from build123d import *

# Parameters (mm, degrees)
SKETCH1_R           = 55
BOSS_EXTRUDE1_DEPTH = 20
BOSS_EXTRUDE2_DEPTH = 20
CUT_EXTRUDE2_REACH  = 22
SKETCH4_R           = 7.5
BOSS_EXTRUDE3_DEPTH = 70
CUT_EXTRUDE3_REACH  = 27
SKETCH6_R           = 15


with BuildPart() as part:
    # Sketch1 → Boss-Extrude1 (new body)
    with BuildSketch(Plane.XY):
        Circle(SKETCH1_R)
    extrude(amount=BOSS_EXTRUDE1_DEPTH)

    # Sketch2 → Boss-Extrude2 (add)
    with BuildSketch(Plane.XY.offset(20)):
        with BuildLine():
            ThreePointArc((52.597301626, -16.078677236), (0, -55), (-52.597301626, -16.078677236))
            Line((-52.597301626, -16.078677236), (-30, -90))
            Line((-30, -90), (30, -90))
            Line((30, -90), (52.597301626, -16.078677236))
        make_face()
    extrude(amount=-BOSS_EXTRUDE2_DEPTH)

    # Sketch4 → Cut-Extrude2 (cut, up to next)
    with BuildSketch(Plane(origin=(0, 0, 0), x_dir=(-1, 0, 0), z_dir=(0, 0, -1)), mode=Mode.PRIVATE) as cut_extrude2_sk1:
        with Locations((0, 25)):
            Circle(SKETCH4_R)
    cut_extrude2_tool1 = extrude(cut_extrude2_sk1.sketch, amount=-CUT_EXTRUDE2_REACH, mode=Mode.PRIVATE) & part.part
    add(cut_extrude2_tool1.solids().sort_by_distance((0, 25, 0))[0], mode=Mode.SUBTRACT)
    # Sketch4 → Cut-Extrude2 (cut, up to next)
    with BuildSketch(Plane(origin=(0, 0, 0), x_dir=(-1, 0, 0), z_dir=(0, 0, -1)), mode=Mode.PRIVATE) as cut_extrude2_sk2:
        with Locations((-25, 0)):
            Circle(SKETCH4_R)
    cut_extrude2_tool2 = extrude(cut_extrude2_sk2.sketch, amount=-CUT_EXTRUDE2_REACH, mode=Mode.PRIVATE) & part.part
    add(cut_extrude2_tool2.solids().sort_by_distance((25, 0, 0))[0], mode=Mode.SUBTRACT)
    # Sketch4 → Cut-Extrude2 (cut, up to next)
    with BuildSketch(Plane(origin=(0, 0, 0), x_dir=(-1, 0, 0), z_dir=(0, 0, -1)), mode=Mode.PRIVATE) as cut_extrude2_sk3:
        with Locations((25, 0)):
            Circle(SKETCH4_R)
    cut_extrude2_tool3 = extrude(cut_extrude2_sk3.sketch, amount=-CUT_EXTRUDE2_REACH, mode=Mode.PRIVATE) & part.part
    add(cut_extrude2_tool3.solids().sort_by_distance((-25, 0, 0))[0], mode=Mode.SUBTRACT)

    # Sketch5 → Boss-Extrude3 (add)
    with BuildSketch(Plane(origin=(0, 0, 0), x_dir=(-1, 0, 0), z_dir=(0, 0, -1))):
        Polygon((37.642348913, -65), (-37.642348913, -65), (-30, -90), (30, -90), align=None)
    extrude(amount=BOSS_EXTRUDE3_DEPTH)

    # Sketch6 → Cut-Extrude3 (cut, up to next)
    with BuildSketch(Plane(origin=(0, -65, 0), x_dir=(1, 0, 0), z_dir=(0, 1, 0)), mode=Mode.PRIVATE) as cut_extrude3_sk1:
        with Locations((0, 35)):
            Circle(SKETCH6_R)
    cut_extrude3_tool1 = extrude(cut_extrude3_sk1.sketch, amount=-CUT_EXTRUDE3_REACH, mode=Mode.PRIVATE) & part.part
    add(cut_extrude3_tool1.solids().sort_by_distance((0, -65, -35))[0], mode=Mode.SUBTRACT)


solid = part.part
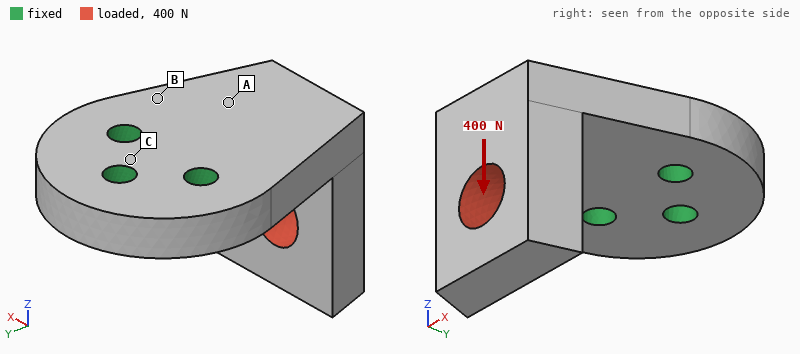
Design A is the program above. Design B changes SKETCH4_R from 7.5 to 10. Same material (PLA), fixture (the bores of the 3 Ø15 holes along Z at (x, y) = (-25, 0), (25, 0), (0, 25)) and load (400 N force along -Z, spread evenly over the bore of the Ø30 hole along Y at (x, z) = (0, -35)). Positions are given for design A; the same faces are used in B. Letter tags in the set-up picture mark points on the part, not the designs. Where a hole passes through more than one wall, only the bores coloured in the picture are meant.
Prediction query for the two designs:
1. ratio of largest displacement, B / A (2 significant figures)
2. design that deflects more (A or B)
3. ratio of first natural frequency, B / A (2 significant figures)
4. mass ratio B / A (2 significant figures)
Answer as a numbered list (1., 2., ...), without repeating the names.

1. 0.91
2. A
3. 1.0
4. 0.98
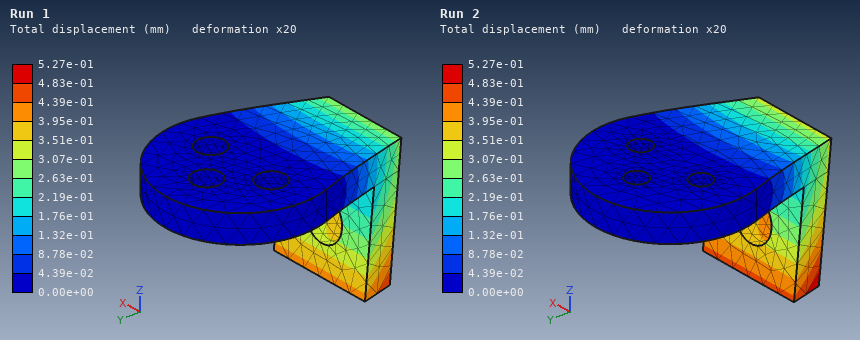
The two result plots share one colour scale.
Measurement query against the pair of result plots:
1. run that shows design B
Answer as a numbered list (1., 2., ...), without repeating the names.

1. Run 1
